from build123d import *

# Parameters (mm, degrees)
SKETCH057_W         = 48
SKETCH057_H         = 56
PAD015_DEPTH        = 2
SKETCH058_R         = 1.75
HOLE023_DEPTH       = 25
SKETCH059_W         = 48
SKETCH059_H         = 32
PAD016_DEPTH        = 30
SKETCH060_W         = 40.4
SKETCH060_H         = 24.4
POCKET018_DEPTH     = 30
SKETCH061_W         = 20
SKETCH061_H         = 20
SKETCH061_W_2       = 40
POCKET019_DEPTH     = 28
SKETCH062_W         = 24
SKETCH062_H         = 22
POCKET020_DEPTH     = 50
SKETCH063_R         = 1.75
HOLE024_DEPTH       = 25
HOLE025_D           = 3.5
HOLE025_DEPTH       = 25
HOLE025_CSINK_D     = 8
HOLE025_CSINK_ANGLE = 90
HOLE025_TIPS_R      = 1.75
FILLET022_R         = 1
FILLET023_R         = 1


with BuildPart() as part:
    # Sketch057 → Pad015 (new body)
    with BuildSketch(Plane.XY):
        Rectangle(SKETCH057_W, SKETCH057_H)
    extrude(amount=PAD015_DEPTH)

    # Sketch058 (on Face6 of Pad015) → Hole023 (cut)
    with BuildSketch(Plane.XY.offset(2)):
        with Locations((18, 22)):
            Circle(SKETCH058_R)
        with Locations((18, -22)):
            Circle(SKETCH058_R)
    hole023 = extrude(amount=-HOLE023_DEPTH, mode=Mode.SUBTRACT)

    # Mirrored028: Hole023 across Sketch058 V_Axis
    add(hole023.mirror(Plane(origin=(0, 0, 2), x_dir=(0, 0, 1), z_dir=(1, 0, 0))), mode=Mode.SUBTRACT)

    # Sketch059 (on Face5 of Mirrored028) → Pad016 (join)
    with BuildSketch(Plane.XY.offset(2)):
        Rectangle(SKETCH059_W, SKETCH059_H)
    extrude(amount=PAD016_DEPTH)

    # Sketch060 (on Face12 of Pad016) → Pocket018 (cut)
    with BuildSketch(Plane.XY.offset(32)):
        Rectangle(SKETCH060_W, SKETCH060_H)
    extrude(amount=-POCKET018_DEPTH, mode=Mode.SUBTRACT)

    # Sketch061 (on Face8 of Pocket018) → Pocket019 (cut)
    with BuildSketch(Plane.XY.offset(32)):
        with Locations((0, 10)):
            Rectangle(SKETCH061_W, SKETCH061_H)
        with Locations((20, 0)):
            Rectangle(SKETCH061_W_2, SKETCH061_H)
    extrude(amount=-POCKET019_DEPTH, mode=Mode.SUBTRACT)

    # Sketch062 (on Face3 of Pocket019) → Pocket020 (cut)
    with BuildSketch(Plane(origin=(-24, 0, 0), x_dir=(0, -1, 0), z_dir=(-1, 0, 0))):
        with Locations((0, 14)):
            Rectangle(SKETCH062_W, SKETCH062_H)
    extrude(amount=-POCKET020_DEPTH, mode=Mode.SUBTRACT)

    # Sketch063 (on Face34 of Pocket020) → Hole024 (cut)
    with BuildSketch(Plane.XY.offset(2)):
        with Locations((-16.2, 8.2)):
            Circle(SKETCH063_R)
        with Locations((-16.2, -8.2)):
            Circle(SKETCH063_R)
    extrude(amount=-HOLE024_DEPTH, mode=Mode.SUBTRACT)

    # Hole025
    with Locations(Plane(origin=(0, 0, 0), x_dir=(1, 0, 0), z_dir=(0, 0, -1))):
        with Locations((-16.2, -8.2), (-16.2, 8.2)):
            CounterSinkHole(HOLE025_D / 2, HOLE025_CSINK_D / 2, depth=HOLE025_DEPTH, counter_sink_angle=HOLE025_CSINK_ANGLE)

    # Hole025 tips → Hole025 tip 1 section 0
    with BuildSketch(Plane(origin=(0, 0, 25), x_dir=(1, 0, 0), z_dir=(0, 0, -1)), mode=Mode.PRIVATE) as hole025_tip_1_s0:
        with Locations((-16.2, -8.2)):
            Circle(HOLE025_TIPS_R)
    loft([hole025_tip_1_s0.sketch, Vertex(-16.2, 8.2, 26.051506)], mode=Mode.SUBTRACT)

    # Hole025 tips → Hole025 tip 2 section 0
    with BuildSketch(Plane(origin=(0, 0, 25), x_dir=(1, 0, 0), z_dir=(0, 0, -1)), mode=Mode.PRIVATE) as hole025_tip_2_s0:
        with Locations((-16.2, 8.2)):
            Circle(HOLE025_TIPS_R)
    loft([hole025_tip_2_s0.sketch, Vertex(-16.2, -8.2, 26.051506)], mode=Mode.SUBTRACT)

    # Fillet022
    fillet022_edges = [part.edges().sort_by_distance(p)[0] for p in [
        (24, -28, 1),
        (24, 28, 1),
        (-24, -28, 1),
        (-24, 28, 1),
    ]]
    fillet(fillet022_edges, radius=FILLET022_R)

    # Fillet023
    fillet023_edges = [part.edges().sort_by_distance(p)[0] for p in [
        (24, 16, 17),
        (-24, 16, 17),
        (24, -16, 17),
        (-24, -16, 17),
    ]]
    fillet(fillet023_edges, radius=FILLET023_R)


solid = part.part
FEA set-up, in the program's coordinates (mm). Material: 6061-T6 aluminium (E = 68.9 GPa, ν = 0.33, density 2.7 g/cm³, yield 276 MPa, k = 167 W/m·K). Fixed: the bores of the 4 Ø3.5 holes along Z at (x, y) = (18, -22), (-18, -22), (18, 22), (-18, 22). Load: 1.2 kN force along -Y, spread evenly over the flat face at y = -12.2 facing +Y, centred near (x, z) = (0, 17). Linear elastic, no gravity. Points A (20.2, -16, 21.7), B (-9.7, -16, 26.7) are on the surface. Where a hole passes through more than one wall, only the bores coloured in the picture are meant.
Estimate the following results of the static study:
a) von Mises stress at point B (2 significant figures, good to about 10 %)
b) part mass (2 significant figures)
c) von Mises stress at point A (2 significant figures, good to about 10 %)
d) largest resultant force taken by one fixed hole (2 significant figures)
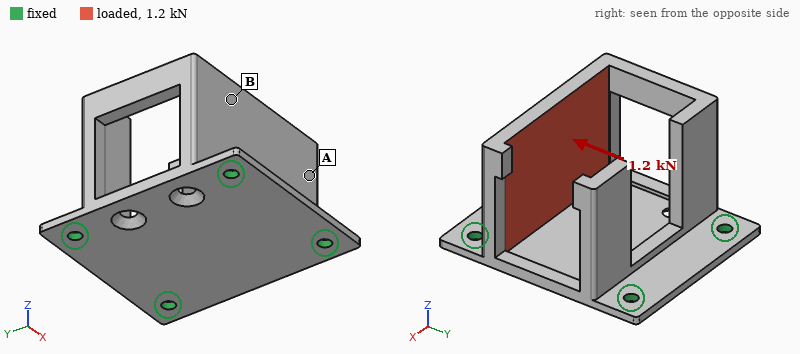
82 MPa
40 g
26 MPa
490 N
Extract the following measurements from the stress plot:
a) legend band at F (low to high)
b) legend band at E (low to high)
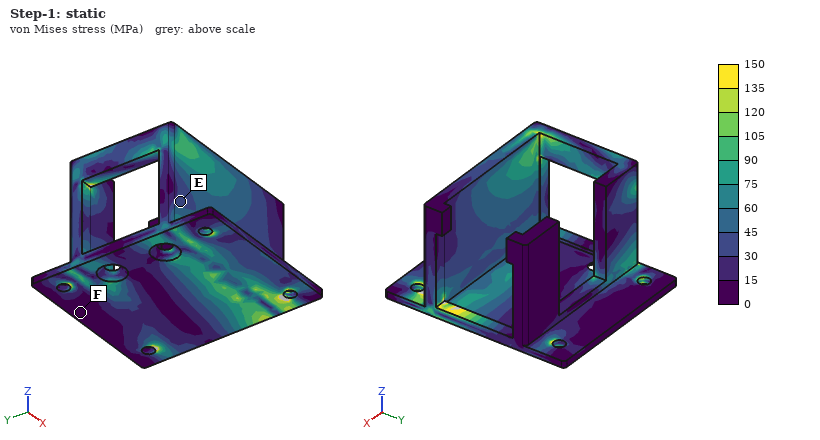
0 to 15 MPa
30 to 45 MPa
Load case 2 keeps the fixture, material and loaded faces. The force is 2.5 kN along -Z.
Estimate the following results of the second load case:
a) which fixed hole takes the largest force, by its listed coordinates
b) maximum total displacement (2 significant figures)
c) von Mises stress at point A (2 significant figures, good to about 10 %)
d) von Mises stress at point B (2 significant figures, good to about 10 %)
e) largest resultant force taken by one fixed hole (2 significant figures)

(18, -22)
0.34 mm
23 MPa
54 MPa
1.2 kN
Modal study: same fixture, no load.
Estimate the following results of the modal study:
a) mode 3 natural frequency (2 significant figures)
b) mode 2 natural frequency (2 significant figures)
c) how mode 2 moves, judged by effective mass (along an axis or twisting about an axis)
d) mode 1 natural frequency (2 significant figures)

3300 Hz
2600 Hz
along Y
2000 Hz
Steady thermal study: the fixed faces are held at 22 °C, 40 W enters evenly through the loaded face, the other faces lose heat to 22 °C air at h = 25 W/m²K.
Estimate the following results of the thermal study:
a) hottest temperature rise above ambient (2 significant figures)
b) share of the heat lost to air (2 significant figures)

38 K
9.4 %
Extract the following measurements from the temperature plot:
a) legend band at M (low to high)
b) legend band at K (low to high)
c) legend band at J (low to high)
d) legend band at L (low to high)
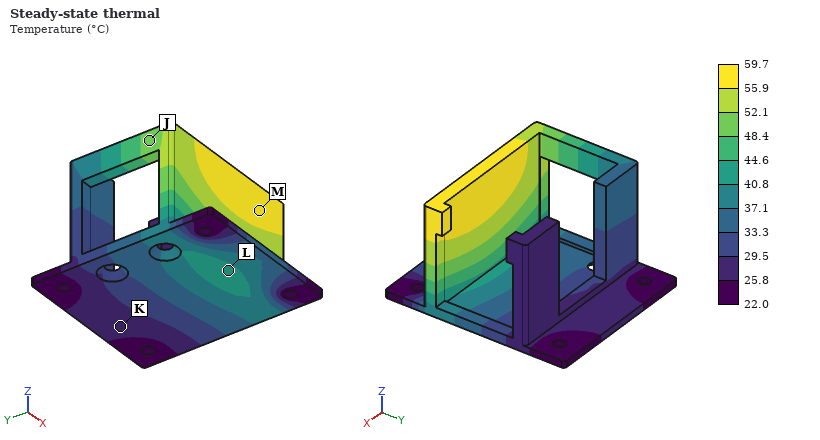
55.9 to 59.7 °C
25.8 to 29.5 °C
48.4 to 52.1 °C
40.8 to 44.6 °C
